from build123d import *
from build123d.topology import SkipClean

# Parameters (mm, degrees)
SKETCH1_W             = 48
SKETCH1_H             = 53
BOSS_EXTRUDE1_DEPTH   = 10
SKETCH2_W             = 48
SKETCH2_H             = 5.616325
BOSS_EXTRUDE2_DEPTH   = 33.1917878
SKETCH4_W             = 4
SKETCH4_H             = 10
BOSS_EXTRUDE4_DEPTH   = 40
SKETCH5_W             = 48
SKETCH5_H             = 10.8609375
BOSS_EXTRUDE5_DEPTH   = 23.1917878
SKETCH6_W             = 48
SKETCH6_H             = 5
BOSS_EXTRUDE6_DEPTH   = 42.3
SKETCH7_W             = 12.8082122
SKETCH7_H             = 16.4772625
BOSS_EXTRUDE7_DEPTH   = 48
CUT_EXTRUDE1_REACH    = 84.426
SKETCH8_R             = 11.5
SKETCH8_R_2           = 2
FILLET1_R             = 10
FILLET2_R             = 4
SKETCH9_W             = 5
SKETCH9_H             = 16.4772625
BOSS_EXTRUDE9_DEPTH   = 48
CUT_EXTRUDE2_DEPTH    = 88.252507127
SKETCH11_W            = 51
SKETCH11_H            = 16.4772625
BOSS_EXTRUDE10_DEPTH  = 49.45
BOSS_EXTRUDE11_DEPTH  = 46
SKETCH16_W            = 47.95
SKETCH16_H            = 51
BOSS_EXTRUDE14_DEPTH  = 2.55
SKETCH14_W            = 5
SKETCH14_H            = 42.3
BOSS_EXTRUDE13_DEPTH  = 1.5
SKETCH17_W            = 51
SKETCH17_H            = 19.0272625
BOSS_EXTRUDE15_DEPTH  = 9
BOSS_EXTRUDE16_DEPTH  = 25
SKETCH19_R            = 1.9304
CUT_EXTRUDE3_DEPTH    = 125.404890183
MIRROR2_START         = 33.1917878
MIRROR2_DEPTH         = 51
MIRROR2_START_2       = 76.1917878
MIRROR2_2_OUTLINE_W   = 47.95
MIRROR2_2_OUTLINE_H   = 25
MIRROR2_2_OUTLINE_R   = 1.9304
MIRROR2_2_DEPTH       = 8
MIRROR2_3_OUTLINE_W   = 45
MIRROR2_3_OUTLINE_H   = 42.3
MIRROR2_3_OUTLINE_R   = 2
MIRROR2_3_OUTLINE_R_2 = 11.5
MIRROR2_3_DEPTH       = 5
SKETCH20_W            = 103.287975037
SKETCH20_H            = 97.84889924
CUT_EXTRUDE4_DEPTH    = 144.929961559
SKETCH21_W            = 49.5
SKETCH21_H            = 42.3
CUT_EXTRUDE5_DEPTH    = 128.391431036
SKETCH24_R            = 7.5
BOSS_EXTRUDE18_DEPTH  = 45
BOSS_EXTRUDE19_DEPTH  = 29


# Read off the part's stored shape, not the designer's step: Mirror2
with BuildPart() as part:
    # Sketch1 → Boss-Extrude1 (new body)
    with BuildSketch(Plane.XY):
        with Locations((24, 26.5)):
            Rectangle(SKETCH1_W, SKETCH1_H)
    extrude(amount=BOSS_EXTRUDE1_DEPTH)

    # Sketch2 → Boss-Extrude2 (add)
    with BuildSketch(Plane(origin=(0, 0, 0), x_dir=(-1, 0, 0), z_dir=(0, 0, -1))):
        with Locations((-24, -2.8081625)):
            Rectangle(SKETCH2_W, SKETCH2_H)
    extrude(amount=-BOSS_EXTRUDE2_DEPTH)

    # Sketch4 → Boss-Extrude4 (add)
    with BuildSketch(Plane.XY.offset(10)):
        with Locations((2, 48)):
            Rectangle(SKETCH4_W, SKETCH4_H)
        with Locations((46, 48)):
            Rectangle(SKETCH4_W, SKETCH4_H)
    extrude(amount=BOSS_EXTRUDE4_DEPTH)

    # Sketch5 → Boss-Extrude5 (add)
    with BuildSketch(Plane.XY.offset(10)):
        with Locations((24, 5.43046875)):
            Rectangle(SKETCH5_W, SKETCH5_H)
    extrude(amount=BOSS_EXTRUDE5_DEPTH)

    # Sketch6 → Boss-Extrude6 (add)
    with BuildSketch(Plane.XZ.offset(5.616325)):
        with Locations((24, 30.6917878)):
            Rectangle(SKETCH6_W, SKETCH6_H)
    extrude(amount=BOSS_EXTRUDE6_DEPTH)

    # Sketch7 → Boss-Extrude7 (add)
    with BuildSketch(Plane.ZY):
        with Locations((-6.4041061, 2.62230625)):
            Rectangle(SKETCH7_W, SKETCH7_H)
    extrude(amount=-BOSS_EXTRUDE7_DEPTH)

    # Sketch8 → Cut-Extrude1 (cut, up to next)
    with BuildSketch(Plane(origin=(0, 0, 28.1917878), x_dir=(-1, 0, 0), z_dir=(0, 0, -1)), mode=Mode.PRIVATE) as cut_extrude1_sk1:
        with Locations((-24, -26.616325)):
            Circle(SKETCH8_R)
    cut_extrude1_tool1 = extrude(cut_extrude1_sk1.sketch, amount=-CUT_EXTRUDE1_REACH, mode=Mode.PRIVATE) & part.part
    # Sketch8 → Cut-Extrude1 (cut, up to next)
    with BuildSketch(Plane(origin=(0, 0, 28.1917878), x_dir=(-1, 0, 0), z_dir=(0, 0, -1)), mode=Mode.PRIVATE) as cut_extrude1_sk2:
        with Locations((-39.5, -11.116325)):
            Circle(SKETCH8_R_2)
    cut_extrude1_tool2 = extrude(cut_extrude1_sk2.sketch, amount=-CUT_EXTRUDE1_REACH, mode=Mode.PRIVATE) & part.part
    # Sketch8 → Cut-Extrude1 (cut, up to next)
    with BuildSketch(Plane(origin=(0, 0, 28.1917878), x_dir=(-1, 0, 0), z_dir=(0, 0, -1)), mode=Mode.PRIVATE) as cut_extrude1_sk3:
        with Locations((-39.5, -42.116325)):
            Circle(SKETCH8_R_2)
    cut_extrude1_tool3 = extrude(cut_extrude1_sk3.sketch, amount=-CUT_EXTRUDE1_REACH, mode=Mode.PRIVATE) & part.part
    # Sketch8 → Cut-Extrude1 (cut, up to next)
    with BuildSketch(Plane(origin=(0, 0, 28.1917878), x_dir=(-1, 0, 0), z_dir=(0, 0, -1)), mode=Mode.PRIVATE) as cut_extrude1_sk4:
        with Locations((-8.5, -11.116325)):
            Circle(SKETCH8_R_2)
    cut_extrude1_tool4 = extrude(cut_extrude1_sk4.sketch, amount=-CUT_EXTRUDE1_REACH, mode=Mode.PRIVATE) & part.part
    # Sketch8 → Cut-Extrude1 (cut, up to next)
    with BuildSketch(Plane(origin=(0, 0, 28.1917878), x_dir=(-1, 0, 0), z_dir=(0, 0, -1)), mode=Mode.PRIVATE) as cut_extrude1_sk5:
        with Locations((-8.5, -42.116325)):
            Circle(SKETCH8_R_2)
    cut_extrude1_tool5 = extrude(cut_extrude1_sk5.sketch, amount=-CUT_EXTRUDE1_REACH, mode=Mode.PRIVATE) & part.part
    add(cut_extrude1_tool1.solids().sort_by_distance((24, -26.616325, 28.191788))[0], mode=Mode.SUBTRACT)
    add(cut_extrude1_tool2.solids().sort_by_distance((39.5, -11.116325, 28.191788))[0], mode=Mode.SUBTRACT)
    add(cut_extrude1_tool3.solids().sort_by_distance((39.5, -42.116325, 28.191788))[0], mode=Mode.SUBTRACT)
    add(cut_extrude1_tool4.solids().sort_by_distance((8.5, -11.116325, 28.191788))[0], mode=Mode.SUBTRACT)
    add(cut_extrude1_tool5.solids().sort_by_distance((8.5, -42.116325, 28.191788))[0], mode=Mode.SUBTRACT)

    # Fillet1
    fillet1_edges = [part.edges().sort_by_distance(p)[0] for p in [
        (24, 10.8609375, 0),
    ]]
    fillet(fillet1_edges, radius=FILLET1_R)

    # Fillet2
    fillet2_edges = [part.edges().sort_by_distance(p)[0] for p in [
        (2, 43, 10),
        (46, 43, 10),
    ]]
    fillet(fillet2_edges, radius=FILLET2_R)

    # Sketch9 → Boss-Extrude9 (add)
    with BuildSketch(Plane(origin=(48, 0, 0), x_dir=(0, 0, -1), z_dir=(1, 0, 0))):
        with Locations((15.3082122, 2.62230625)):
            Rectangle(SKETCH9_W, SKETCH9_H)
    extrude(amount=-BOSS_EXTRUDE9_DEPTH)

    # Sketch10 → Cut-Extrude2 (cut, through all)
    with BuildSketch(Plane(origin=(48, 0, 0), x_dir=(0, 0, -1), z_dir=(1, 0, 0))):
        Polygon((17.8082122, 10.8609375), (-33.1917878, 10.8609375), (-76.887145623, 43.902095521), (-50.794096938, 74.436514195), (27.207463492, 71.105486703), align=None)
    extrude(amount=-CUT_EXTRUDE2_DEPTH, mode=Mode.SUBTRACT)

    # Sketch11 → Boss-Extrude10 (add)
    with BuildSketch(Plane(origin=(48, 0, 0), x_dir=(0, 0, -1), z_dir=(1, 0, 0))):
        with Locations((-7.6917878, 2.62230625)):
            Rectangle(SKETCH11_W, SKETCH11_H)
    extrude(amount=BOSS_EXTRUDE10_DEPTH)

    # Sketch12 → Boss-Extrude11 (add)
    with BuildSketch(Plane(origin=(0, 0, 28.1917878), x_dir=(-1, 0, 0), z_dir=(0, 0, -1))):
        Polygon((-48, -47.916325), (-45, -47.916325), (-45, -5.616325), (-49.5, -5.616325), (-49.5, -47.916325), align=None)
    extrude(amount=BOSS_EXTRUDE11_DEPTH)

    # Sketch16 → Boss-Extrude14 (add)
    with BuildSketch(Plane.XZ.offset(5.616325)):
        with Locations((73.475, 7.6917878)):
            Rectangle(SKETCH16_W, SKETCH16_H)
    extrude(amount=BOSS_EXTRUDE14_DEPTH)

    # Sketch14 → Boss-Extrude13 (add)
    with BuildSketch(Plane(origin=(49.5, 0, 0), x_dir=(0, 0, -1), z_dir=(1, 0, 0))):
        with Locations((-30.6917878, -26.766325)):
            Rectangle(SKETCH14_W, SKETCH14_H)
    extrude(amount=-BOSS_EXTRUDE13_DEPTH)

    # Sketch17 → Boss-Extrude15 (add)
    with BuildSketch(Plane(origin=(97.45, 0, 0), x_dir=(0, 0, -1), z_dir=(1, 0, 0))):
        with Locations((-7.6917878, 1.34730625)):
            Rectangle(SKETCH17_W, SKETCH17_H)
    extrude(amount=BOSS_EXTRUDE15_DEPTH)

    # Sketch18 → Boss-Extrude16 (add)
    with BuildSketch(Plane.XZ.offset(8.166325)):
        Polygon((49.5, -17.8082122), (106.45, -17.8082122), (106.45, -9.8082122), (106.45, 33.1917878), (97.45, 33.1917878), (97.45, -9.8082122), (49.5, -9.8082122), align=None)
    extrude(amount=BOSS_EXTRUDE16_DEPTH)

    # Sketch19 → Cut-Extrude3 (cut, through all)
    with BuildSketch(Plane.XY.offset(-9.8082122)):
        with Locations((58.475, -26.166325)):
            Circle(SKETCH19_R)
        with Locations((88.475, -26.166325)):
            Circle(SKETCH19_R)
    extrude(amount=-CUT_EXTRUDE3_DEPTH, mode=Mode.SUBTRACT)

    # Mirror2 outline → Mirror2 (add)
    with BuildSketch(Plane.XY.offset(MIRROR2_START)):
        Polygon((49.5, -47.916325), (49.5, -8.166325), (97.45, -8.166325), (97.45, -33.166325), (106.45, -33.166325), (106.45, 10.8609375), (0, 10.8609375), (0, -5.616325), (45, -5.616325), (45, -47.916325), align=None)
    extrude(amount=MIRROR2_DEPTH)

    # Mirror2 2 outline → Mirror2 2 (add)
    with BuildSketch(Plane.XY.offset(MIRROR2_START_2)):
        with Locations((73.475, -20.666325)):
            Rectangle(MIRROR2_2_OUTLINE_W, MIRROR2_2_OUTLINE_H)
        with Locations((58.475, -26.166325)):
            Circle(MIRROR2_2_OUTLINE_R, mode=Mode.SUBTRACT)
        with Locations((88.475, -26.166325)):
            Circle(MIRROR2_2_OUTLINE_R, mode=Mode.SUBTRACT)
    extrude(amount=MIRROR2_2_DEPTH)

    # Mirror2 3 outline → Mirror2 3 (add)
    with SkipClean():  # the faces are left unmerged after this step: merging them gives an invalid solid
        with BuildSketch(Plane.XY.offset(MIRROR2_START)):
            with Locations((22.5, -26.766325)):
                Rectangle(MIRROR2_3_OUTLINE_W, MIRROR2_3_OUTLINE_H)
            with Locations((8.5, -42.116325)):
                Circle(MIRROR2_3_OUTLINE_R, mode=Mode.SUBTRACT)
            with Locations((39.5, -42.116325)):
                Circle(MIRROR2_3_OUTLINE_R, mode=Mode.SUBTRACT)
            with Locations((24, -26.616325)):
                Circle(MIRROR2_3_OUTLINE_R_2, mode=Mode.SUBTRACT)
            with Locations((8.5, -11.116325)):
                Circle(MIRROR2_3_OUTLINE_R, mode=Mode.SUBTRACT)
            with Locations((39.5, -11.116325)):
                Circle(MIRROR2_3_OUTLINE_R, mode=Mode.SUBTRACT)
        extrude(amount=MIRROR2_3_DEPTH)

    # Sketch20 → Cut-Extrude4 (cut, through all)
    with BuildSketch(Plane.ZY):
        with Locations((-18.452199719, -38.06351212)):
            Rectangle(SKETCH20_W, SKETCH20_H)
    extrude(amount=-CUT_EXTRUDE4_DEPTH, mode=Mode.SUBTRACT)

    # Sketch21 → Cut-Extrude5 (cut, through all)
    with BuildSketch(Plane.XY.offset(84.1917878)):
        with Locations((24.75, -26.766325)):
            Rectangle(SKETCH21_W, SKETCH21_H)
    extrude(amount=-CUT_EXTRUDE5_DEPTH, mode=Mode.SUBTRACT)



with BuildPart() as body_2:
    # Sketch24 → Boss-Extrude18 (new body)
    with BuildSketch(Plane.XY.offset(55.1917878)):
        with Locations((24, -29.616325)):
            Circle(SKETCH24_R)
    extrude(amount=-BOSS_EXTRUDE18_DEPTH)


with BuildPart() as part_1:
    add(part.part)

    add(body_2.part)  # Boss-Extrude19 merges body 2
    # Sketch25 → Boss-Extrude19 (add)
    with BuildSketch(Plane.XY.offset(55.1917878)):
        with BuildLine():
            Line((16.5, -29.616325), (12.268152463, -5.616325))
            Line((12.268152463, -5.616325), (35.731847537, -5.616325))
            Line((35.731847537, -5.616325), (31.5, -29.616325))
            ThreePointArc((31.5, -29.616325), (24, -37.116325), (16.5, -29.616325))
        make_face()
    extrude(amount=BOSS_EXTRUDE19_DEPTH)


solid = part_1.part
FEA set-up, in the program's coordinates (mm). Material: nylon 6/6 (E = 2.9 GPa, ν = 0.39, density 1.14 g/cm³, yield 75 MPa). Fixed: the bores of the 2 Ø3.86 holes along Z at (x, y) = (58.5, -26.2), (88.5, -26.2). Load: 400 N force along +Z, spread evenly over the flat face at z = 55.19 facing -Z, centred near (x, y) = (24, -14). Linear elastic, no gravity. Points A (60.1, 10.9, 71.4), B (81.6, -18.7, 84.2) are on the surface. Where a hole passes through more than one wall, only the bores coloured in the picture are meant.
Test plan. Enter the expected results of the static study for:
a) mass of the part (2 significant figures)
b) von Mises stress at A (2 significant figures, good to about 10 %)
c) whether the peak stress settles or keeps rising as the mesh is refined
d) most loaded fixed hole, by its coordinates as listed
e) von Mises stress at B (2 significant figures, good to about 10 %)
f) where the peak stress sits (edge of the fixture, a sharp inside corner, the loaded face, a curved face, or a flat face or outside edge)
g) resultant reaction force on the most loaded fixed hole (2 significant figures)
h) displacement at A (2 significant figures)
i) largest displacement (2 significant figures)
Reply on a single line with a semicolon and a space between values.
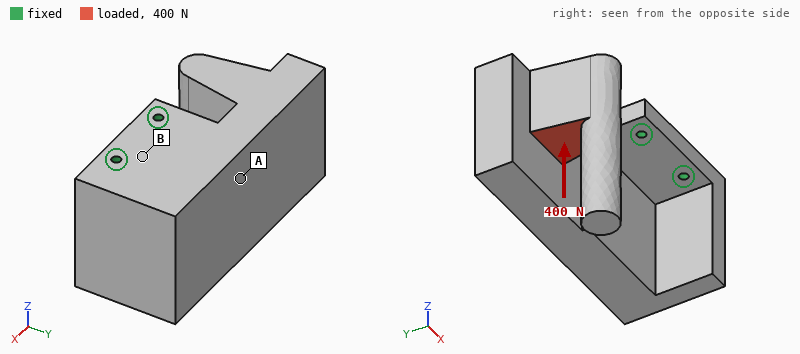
160 g; 2.7 MPa; keeps rising; (58.5, -26.2); 8.9 MPa; edge of the fixture; 730 N; 0.27 mm; 1.5 mm
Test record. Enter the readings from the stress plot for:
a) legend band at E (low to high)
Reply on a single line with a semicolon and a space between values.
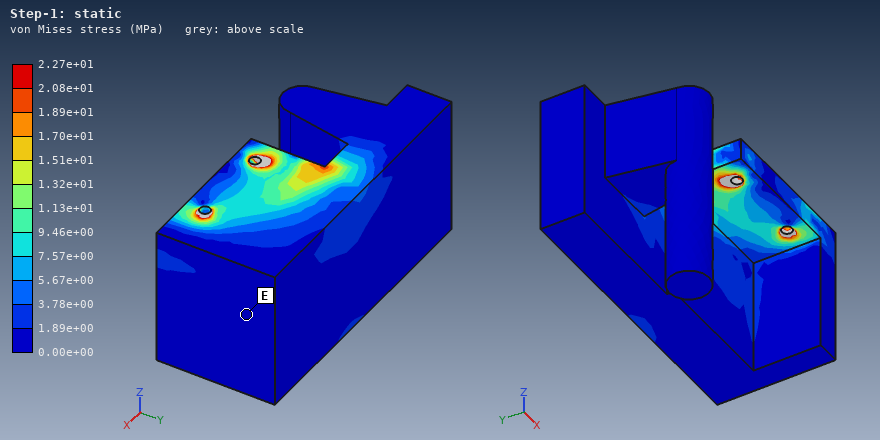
0.00e+00 to 1.89e+00 MPa
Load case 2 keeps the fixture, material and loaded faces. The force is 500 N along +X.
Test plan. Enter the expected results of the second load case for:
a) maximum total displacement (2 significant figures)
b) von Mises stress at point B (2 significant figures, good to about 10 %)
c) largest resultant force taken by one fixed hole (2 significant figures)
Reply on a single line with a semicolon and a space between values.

1.2 mm; 4.3 MPa; 450 N
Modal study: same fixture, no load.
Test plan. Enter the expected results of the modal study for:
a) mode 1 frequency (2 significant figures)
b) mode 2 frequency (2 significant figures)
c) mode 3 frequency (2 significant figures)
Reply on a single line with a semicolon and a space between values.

250 Hz; 330 Hz; 600 Hz
